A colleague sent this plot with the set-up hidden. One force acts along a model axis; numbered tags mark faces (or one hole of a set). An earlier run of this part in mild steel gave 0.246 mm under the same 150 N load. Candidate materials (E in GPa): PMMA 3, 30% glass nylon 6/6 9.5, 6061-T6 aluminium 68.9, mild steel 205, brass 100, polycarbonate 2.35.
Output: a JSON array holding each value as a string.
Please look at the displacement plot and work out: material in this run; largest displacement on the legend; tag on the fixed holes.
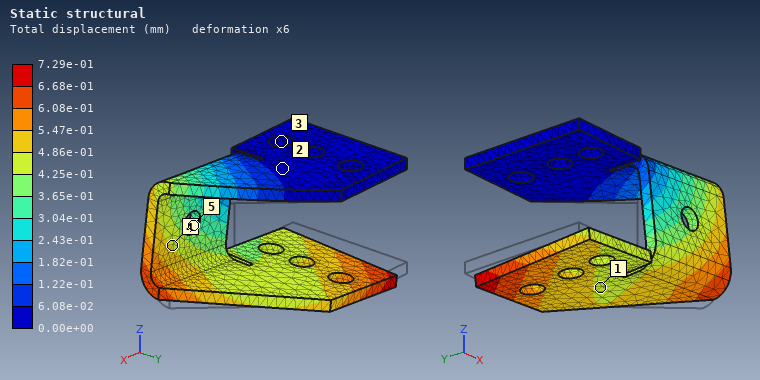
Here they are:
["6061-T6 aluminium", "7.29e-01 mm", "3"]
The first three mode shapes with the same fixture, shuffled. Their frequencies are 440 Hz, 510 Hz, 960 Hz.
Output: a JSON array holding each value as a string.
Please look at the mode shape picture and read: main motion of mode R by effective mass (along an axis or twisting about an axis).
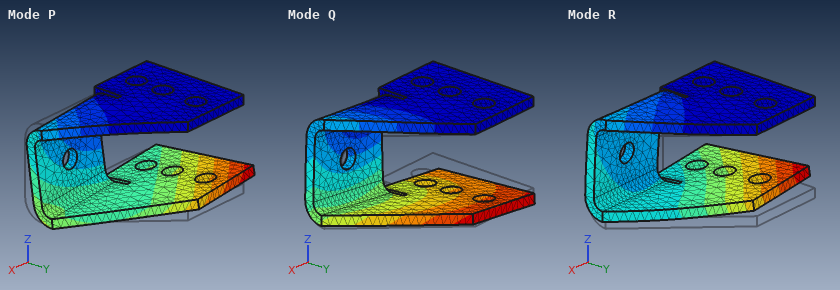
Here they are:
["along Z"]
